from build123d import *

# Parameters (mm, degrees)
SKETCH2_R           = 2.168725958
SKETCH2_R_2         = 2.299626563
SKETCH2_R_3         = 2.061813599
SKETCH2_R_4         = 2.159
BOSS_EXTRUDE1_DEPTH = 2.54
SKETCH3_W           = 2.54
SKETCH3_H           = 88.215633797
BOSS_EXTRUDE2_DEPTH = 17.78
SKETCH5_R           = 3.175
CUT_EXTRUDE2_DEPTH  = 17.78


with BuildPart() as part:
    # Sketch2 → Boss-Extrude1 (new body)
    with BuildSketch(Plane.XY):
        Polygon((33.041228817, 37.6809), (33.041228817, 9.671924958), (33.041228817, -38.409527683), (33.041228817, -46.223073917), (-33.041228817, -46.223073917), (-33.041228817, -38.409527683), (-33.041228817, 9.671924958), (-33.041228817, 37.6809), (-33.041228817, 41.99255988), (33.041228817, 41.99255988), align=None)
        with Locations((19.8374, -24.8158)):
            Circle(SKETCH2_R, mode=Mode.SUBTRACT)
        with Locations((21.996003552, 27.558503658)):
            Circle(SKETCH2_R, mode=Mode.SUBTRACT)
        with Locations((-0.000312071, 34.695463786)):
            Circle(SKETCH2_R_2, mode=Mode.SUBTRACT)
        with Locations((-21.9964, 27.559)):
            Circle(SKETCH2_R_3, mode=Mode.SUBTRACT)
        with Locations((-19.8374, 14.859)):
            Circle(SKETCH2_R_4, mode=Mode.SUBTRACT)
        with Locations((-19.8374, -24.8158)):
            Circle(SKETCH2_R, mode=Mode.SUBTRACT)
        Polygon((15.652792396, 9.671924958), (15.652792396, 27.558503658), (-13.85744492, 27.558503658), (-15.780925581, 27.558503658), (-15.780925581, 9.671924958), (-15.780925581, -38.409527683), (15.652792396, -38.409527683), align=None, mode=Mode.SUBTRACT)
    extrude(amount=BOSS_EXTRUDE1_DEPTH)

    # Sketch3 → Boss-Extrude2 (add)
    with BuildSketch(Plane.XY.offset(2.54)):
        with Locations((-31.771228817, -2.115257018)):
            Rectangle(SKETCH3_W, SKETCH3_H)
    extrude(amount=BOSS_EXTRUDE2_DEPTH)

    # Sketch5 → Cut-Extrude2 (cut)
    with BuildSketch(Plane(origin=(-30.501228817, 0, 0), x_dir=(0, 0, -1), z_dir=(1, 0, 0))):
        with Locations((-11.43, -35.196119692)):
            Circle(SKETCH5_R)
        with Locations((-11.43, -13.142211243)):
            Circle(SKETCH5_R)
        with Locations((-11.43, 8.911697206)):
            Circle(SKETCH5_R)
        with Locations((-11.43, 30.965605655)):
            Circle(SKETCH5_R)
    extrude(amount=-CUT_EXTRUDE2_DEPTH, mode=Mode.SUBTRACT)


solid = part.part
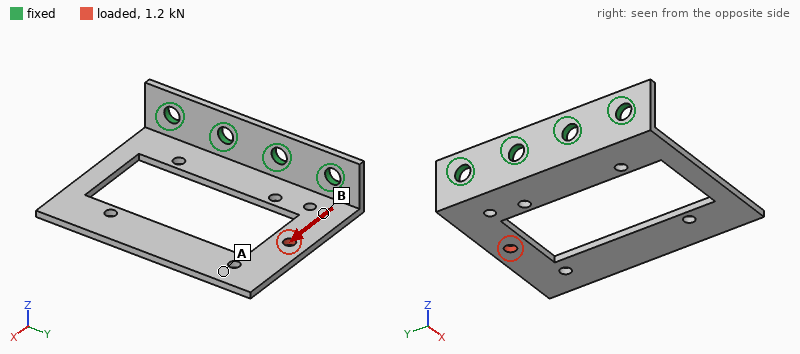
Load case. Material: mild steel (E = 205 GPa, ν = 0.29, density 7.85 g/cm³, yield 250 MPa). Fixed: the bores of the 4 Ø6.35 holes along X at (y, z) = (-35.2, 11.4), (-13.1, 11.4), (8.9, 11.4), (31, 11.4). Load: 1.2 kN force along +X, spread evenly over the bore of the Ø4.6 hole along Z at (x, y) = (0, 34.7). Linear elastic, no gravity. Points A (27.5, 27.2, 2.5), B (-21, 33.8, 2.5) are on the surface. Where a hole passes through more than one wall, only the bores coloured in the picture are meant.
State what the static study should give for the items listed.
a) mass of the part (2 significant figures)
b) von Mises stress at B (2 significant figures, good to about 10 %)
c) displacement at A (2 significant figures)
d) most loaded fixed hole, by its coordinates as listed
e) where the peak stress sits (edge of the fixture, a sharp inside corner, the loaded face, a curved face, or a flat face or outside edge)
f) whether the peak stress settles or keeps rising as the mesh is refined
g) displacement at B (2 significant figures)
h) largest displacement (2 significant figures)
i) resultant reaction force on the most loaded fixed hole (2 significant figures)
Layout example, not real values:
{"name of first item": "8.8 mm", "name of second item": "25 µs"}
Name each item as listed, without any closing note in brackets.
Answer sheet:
{"mass of the part": "100 g", "von Mises stress at B": "49 MPa", "displacement at A": "0.19 mm", "most loaded fixed hole, by its coordinates as listed": "(31, 11.4)", "where the peak stress sits": "edge of the fixture", "whether the peak stress settles or keeps rising as the mesh is refined": "keeps rising", "displacement at B": "0.056 mm", "largest displacement": "0.24 mm", "resultant reaction force on the most loaded fixed hole": "1.0 kN"}
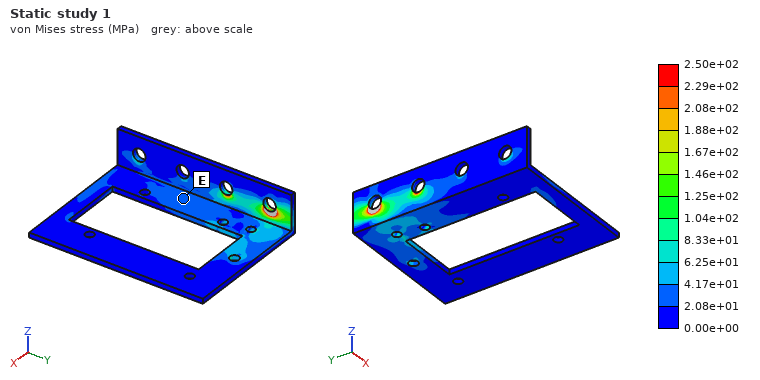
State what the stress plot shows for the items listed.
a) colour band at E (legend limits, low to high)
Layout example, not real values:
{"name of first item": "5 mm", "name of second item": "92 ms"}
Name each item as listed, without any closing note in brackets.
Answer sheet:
{"colour band at E": "2.08e+01 to 4.17e+01 MPa"}
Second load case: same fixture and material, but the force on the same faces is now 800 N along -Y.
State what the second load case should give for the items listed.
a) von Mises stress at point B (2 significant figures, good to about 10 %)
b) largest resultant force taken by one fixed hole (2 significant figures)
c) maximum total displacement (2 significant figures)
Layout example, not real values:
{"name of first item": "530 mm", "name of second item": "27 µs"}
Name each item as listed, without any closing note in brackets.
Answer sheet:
{"von Mises stress at point B": "22 MPa", "largest resultant force taken by one fixed hole": "430 N", "maximum total displacement": "96 µm"}
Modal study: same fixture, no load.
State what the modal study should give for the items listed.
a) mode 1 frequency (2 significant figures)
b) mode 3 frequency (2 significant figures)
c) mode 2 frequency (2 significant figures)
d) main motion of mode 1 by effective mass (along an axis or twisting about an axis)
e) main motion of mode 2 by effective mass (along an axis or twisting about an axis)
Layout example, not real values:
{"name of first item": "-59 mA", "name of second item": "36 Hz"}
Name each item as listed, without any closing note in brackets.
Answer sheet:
{"mode 1 frequency": "300 Hz", "mode 3 frequency": "1900 Hz", "mode 2 frequency": "710 Hz", "main motion of mode 1 by effective mass": "along Z", "main motion of mode 2 by effective mass": "twisting about X"}
